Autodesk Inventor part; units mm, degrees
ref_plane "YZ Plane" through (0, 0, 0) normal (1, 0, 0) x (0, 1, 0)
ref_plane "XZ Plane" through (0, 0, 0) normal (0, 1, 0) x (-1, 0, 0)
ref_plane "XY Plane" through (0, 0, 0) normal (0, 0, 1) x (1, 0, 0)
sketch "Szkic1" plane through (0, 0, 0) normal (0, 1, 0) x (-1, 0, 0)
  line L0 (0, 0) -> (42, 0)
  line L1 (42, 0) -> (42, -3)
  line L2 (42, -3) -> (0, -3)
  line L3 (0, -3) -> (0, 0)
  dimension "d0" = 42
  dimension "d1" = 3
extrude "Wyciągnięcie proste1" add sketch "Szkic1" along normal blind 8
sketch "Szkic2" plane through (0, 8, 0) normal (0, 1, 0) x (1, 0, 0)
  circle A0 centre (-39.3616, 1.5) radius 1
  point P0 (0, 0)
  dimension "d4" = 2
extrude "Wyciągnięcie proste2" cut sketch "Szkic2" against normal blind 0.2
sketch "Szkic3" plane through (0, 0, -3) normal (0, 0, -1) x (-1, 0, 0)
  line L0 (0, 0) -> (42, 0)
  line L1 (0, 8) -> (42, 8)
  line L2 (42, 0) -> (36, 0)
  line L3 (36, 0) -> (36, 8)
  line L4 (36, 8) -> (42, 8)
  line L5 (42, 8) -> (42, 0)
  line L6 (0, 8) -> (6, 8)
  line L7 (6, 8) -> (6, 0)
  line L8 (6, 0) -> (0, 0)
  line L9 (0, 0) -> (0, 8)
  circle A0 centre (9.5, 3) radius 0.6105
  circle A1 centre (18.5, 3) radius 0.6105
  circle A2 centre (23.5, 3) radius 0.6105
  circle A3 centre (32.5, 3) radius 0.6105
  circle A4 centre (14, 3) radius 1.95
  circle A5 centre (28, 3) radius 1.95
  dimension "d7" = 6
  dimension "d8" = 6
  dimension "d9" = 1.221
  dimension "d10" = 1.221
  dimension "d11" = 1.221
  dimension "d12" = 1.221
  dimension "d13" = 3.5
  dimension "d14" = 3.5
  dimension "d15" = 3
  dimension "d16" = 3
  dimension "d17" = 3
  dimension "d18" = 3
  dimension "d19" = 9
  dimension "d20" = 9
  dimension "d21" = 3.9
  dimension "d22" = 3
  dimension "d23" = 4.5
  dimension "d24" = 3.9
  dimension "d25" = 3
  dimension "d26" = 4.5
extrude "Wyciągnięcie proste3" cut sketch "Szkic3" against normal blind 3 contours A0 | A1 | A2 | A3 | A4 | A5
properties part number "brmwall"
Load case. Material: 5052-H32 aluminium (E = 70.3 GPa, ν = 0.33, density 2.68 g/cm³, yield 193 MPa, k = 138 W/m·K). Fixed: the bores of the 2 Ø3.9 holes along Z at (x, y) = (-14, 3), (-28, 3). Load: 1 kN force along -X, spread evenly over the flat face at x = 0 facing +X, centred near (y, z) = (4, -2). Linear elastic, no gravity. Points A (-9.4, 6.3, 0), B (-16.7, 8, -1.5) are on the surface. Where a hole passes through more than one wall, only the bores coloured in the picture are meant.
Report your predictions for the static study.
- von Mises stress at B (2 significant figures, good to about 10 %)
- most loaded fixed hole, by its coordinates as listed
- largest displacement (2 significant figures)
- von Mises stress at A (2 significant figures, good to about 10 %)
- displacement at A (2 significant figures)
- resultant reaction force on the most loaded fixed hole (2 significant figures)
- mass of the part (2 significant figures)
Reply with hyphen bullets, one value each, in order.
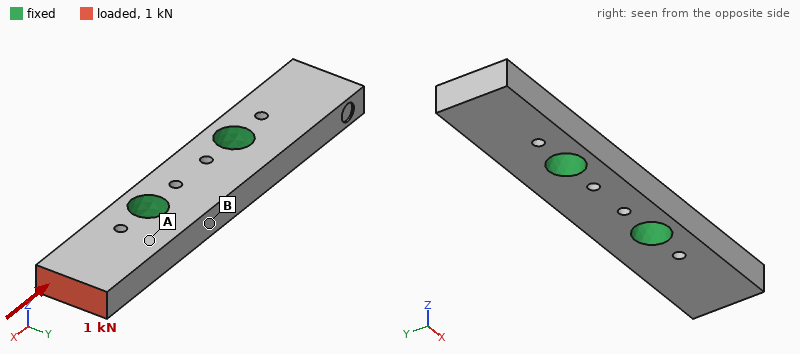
- 17 MPa
- (-14, 3)
- 10 µm
- 40 MPa
- 3.9 µm
- 950 N
- 2.5 g
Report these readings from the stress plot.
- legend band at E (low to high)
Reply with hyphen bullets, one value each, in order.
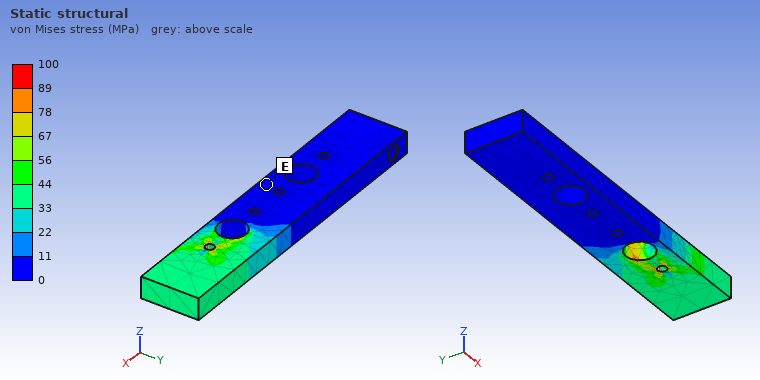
- 0 to 11 MPa
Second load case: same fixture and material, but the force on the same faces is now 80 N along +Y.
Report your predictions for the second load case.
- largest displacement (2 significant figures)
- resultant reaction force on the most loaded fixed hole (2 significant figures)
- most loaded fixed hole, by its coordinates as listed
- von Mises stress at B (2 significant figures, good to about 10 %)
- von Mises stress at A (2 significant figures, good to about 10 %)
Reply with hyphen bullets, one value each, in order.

- 12 µm
- 100 N
- (-14, 3)
- 9.5 MPa
- 14 MPa
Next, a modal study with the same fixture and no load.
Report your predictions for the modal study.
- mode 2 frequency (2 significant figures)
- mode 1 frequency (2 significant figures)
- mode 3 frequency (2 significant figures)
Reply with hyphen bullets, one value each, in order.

- 14 kHz
- 14 kHz
- 27 kHz
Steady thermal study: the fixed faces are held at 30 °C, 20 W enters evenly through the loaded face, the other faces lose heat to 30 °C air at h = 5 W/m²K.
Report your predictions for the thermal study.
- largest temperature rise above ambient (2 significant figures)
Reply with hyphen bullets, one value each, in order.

- 80 K
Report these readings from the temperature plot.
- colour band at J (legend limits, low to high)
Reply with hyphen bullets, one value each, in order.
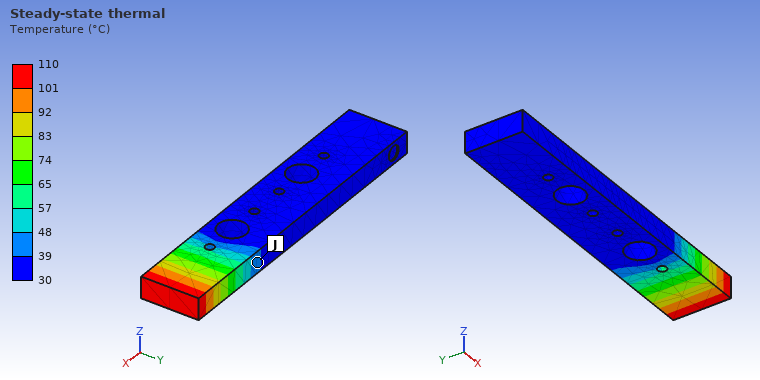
- 39 to 48 °C
